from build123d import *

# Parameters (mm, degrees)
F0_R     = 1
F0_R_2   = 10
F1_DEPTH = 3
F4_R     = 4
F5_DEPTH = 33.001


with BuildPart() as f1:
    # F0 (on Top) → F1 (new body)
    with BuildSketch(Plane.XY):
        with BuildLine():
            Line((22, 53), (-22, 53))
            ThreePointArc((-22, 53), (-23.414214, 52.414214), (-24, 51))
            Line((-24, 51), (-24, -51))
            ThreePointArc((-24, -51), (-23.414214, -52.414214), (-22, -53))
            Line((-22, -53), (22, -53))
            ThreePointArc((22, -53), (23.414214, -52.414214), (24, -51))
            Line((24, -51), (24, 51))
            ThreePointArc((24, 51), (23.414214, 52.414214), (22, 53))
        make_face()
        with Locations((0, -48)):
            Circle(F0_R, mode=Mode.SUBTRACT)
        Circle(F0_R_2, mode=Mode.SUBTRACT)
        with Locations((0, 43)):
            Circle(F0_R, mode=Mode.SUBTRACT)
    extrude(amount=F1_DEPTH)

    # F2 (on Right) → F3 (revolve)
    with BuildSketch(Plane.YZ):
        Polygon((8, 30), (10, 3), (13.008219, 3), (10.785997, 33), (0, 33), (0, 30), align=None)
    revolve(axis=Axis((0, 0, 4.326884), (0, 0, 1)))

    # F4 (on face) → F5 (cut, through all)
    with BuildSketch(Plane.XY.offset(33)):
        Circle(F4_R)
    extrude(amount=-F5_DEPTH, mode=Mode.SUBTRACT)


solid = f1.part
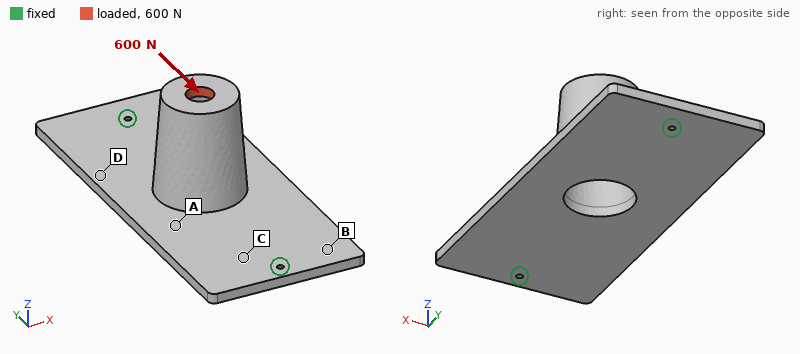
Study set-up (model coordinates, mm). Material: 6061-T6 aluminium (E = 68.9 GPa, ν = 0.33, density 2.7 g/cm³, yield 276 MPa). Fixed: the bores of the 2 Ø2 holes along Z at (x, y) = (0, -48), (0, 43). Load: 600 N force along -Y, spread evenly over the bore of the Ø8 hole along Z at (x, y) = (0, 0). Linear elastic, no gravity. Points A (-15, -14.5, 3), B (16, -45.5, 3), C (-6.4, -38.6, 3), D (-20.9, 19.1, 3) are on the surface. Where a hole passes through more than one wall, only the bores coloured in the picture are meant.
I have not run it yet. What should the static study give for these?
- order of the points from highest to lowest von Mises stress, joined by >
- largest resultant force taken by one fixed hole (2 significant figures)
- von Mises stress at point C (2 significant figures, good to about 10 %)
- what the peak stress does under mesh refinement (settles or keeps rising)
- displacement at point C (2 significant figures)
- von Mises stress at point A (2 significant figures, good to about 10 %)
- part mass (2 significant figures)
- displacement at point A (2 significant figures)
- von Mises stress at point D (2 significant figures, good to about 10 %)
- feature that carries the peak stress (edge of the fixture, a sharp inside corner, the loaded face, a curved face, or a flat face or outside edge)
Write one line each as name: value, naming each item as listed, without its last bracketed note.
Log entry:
order of the points from highest to lowest von Mises stress, joined by >: A > D > C > B
largest resultant force taken by one fixed hole: 400 N
von Mises stress at point C: 18 MPa
what the peak stress does under mesh refinement: keeps rising
displacement at point C: 0.049 mm
von Mises stress at point A: 59 MPa
part mass: 56 g
displacement at point A: 0.12 mm
von Mises stress at point D: 44 MPa
feature that carries the peak stress: edge of the fixture
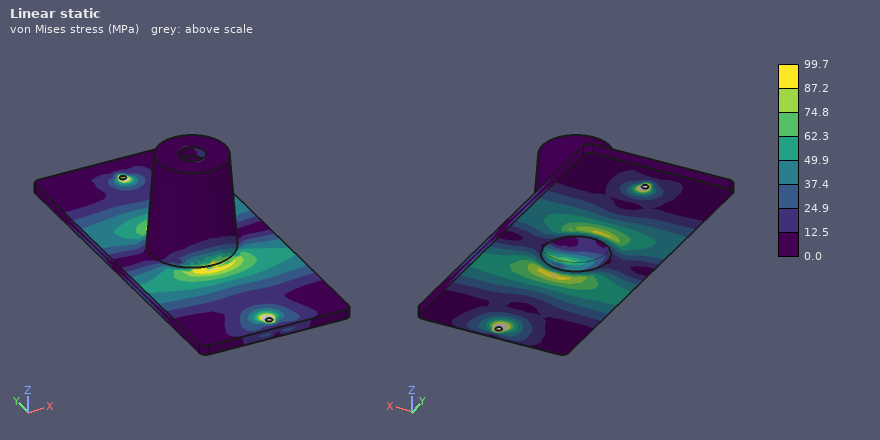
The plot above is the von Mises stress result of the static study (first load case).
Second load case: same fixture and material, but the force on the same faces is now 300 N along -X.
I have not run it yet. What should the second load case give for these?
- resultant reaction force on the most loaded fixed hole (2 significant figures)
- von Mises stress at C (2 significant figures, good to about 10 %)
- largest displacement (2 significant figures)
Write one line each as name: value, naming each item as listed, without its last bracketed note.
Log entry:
resultant reaction force on the most loaded fixed hole: 160 N
von Mises stress at C: 56 MPa
largest displacement: 0.66 mm
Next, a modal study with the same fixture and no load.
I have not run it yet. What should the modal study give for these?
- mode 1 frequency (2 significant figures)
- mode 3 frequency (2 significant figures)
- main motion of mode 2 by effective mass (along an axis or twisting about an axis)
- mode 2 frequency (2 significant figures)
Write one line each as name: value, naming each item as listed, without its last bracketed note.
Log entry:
mode 1 frequency: 1000 Hz
mode 3 frequency: 2400 Hz
main motion of mode 2 by effective mass: along Z
mode 2 frequency: 1200 Hz
